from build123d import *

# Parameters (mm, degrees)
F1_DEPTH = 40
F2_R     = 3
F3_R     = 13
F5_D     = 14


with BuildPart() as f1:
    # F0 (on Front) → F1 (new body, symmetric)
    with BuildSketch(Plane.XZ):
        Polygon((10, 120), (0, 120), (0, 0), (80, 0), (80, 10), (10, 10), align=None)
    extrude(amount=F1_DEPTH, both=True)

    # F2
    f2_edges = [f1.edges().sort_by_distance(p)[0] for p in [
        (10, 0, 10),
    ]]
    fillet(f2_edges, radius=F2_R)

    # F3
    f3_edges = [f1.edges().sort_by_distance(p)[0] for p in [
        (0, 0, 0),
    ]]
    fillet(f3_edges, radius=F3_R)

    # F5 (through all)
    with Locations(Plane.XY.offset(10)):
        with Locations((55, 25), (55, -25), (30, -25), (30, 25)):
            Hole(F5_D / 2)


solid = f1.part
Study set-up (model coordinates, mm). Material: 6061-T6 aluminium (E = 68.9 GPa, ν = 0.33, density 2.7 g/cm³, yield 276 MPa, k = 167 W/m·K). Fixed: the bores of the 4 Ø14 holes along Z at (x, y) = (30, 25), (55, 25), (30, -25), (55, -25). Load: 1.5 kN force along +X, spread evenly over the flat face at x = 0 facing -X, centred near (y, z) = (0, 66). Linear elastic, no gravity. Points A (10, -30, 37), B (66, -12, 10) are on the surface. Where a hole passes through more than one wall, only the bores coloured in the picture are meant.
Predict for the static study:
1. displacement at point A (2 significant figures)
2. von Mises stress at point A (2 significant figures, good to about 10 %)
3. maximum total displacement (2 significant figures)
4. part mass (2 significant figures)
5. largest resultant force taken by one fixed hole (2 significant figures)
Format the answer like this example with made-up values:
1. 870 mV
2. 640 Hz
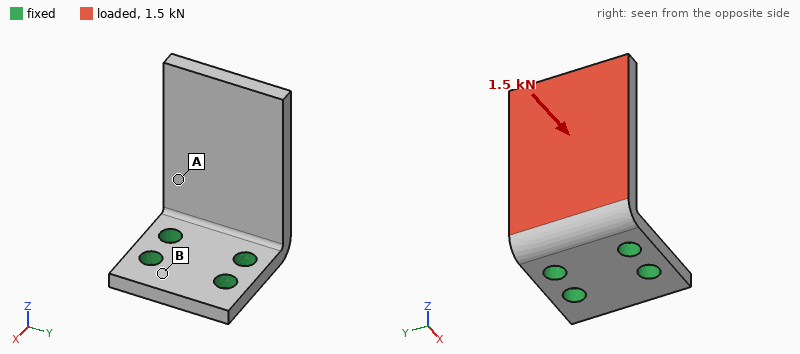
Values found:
1. 0.18 mm
2. 35 MPa
3. 1.0 mm
4. 390 g
5. 720 N
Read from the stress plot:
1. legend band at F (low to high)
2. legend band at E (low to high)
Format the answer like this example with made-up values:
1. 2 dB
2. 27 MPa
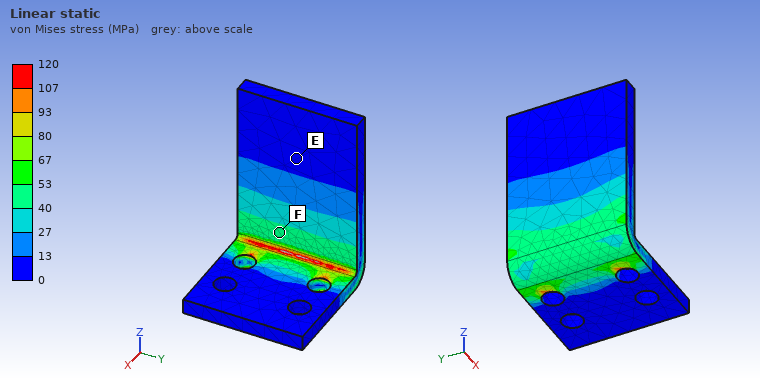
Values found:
1. 40 to 53 MPa
2. 0 to 13 MPa
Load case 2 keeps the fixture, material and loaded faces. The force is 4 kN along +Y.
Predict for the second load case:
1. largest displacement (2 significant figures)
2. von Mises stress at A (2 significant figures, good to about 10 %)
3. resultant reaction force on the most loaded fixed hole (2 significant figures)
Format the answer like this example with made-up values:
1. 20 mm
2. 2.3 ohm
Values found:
1. 0.23 mm
2. 19 MPa
3. 5.2 kN
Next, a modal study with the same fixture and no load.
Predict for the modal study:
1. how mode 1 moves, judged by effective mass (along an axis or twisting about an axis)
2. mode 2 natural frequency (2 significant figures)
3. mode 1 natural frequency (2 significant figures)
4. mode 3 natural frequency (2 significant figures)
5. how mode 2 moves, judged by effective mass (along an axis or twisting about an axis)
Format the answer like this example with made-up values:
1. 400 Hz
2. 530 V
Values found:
1. along X
2. 1500 Hz
3. 490 Hz
4. 2000 Hz
5. along Y
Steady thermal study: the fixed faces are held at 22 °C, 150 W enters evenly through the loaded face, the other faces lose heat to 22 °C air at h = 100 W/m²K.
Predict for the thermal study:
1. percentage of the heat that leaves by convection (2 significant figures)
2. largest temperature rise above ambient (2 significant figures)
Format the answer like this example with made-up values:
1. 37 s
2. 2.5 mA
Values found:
1. 37 %
2. 55 K
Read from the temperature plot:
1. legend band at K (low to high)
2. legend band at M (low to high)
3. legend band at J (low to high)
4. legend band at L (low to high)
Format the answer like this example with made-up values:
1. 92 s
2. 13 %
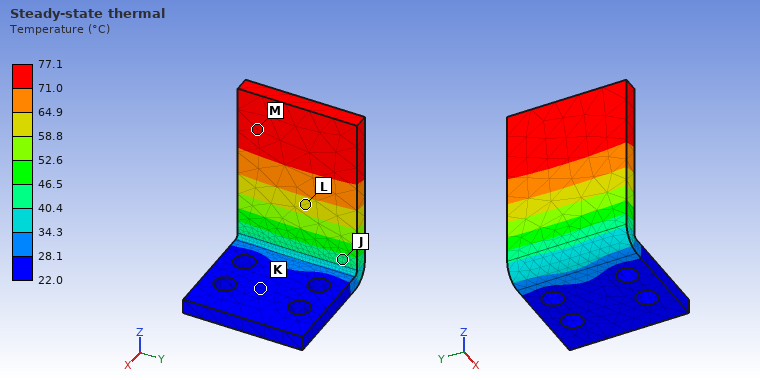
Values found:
1. 22.0 to 28.1 °C
2. 71.0 to 77.1 °C
3. 40.4 to 46.5 °C
4. 58.8 to 64.9 °C
